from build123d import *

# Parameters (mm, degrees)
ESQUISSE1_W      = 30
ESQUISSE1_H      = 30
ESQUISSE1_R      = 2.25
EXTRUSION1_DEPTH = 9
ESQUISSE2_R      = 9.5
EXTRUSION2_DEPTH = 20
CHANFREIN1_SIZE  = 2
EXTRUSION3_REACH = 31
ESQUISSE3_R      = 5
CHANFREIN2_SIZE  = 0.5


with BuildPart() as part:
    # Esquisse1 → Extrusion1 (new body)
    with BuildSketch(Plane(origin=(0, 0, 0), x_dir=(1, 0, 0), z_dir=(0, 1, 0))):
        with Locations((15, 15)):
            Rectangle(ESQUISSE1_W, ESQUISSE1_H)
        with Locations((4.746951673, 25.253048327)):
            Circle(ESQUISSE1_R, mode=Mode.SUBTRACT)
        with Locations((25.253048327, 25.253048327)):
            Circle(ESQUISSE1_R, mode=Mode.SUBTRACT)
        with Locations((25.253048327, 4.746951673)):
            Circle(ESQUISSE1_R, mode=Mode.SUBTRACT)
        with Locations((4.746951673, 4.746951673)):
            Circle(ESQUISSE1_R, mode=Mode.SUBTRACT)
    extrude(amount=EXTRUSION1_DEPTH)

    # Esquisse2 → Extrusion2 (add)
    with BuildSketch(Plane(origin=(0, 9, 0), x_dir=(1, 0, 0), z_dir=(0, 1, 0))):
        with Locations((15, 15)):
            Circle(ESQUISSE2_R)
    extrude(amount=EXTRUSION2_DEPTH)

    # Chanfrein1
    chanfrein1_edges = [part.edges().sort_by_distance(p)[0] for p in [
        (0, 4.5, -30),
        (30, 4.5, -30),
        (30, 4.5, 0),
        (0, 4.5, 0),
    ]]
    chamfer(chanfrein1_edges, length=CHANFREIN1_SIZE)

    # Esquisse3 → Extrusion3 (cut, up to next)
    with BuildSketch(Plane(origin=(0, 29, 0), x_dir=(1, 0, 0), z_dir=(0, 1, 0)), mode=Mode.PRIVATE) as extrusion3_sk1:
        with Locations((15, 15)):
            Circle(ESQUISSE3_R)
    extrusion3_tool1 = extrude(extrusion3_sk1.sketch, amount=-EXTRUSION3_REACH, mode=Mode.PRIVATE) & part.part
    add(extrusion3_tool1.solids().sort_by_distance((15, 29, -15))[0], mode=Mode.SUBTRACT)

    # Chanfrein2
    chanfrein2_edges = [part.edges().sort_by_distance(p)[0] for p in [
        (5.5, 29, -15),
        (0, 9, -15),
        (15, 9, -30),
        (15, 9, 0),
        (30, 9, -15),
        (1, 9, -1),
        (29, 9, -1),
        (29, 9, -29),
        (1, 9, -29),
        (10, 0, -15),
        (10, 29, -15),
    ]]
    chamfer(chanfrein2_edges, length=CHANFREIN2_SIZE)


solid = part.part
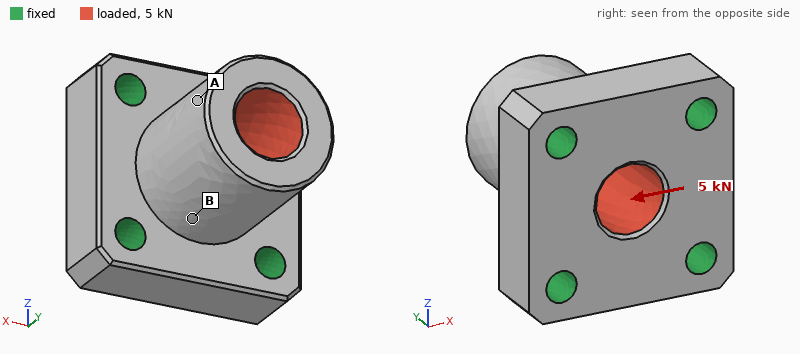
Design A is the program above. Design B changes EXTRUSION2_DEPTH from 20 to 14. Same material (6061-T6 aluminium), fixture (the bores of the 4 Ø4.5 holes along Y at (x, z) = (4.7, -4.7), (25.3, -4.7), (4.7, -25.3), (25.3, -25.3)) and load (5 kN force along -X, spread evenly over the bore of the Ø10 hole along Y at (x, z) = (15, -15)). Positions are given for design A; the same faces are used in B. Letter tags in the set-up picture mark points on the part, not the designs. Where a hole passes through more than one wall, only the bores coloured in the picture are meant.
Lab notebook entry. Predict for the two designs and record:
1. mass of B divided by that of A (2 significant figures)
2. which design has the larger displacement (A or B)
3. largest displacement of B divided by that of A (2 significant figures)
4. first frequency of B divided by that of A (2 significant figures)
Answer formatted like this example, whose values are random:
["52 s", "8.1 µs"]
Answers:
["0.89", "A", "0.52", "1.5"]
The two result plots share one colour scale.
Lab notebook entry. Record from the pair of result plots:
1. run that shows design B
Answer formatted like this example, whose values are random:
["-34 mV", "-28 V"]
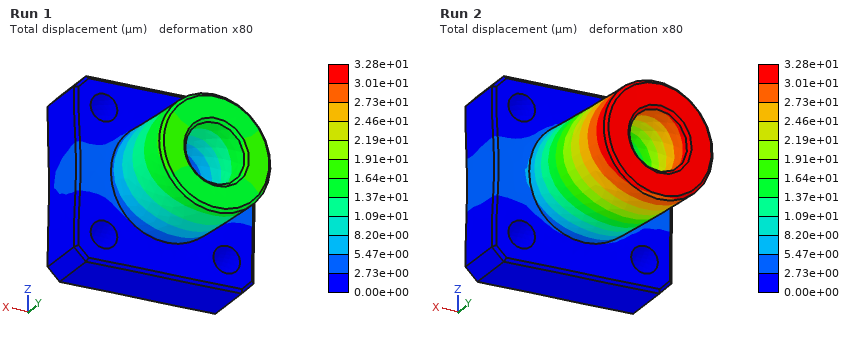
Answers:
["Run 1"]
